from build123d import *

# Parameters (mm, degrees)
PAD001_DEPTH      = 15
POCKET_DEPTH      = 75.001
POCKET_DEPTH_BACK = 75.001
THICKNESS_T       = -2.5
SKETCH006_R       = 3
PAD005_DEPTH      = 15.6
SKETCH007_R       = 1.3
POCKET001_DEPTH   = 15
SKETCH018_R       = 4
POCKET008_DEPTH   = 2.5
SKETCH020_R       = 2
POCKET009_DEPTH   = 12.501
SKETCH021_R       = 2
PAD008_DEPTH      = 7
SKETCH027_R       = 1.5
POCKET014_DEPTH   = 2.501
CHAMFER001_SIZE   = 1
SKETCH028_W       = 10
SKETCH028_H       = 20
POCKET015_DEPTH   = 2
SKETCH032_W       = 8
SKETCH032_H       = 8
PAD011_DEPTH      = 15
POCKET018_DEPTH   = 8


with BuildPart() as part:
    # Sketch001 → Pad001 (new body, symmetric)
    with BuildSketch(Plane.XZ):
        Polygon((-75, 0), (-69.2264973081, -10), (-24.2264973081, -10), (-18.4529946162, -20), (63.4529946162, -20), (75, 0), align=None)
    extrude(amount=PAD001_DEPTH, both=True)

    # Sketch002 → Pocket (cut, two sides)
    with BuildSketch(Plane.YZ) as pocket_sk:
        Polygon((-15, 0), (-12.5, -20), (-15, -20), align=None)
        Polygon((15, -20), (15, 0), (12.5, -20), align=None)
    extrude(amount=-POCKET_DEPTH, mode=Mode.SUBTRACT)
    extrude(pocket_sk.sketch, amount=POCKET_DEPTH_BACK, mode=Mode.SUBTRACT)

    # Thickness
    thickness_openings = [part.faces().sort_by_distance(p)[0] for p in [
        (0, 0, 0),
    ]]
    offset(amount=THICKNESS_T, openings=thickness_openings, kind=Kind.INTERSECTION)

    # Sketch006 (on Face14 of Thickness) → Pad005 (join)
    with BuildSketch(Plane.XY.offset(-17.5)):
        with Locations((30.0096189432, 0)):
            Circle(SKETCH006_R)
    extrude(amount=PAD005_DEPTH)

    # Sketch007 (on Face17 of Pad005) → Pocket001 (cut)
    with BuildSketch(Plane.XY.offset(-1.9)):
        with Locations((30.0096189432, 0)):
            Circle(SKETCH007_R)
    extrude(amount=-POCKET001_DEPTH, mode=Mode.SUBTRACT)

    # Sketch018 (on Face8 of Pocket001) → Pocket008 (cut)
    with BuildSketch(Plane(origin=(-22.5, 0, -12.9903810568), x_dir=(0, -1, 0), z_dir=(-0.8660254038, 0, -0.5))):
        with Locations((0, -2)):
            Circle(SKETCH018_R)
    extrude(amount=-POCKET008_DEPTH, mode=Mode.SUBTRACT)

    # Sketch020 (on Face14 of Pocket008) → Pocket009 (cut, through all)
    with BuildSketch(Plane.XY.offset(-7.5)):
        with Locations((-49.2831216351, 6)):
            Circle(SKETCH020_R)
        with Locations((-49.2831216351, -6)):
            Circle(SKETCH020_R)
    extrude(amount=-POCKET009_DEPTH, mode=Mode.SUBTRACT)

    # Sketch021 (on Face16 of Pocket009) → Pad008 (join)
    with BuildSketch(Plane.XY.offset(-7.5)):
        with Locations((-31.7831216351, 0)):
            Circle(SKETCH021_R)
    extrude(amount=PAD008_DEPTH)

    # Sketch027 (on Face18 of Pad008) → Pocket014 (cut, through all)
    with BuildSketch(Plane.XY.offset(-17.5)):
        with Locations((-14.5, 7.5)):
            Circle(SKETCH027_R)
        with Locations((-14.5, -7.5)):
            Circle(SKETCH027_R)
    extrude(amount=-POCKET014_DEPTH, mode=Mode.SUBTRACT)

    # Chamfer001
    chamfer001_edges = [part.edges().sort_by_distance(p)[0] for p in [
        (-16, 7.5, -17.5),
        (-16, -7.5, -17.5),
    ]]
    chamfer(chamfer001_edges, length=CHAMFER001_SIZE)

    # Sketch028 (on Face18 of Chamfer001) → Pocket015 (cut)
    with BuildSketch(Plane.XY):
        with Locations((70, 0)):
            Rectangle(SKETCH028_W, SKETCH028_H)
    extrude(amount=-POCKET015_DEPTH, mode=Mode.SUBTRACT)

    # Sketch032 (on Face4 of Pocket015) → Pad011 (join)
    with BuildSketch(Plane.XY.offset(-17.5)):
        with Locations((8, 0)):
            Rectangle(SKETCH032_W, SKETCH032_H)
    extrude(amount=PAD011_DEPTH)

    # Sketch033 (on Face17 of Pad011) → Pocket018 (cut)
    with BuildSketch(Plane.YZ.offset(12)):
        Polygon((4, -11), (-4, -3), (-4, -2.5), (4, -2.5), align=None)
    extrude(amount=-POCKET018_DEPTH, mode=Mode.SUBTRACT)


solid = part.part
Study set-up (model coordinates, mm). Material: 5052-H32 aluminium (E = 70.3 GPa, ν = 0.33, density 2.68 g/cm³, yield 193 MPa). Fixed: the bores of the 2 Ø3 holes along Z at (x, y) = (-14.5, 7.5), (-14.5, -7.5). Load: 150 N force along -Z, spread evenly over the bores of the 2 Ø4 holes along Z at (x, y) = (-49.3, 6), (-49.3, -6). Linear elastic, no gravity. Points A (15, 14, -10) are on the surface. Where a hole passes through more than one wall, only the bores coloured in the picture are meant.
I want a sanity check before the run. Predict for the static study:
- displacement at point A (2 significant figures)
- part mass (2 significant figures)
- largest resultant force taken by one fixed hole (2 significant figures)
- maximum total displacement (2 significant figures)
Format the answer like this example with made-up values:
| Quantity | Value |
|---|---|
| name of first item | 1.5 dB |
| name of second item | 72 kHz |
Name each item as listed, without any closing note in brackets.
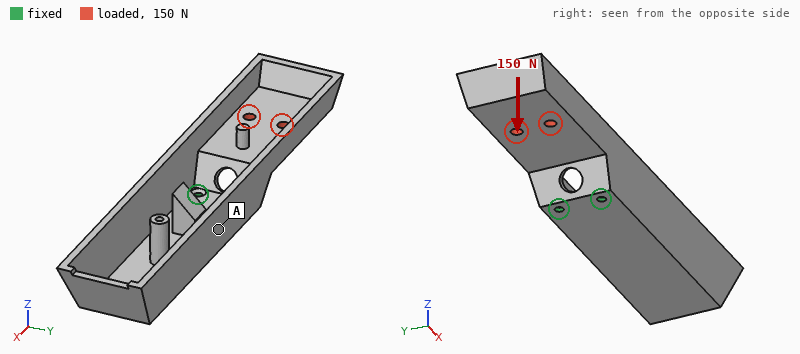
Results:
| Quantity | Value |
|---|---|
| displacement at point A | 0.16 mm |
| part mass | 58 g |
| largest resultant force taken by one fixed hole | 79 N |
| maximum total displacement | 0.46 mm |
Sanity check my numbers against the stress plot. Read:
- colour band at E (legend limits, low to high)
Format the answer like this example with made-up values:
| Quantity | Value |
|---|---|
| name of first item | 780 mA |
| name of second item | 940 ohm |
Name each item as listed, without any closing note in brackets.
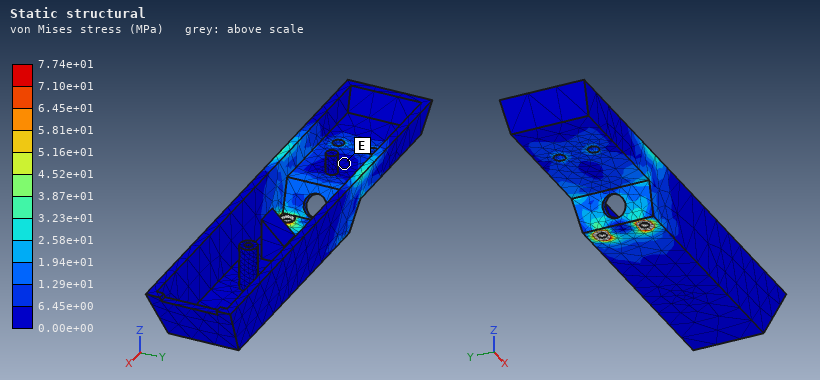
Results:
| Quantity | Value |
|---|---|
| colour band at E | 0.00e+00 to 6.45e+00 MPa |
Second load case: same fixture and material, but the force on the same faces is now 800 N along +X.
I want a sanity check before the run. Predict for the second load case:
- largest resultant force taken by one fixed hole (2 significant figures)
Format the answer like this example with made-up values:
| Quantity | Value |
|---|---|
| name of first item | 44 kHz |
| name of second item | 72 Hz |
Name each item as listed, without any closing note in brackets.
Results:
| Quantity | Value |
|---|---|
| largest resultant force taken by one fixed hole | 410 N |
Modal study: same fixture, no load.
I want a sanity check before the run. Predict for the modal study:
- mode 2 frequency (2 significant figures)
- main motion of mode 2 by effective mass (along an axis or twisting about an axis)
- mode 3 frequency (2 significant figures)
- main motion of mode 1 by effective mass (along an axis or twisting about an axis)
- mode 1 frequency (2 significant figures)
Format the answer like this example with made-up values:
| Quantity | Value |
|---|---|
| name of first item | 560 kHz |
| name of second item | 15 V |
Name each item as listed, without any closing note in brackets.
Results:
| Quantity | Value |
|---|---|
| mode 2 frequency | 1100 Hz |
| main motion of mode 2 by effective mass | along Y |
| mode 3 frequency | 1900 Hz |
| main motion of mode 1 by effective mass | along Z |
| mode 1 frequency | 440 Hz |
